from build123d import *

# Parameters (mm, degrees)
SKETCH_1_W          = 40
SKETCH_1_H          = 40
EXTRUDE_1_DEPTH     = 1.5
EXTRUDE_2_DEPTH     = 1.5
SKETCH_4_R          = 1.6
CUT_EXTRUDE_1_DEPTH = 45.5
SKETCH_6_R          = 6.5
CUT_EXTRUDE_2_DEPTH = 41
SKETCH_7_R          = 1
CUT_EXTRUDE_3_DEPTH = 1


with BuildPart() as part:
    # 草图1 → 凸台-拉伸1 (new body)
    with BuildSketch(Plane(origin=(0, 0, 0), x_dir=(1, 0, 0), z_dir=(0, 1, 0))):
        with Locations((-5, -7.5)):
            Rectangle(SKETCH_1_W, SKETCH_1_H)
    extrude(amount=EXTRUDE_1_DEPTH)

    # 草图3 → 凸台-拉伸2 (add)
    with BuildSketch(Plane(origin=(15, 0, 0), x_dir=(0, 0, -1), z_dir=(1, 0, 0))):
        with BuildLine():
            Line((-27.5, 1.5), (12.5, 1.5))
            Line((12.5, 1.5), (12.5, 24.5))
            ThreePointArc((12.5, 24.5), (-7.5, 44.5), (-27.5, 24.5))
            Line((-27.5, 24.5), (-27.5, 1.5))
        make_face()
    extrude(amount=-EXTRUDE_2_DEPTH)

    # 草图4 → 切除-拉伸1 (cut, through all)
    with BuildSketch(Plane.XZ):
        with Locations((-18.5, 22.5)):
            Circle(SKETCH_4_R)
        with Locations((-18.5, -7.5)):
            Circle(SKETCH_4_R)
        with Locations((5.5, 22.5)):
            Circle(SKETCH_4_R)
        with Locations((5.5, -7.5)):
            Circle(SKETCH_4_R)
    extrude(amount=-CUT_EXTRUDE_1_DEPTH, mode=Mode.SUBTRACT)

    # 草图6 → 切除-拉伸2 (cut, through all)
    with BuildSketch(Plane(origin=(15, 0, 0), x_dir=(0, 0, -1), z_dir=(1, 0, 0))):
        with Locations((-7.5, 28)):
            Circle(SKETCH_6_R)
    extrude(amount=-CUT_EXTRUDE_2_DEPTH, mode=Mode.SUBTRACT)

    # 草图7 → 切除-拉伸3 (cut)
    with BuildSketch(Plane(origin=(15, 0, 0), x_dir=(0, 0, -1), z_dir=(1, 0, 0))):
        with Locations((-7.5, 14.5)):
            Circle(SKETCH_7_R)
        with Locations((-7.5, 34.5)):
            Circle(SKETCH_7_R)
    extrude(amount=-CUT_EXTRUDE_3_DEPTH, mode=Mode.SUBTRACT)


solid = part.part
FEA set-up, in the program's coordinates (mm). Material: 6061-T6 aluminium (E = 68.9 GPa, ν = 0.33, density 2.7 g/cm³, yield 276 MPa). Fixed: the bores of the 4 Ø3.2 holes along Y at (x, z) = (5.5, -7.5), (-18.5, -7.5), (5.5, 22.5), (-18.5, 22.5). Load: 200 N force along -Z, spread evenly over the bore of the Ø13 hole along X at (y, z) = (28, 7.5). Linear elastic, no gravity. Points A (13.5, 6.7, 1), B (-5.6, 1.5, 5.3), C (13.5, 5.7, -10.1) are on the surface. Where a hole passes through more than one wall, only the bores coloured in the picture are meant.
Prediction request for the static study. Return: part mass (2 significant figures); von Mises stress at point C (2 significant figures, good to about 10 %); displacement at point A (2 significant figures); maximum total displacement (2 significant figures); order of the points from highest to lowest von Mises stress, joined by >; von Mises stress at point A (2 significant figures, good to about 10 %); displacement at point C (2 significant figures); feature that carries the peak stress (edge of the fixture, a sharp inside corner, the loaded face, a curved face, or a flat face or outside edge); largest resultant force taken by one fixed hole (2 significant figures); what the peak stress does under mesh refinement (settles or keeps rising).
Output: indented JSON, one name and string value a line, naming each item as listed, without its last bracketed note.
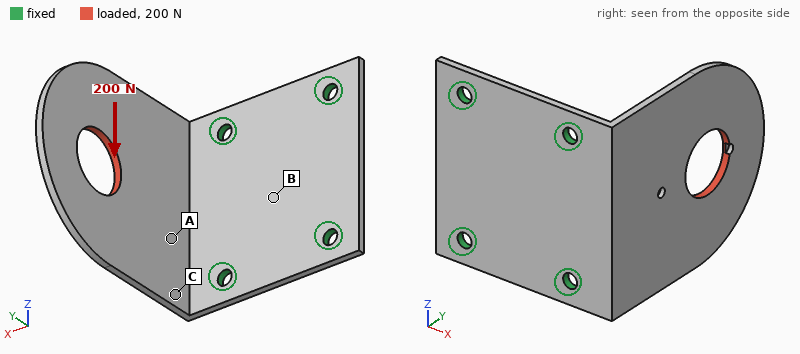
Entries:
{
  "part mass": "12 g",
  "von Mises stress at point C": "62 MPa",
  "displacement at point A": "0.051 mm",
  "maximum total displacement": "0.25 mm",
  "order of the points from highest to lowest von Mises stress, joined by >": "C > A > B",
  "von Mises stress at point A": "38 MPa",
  "displacement at point C": "0.10 mm",
  "feature that carries the peak stress": "edge of the fixture",
  "largest resultant force taken by one fixed hole": "210 N",
  "what the peak stress does under mesh refinement": "keeps rising"
}
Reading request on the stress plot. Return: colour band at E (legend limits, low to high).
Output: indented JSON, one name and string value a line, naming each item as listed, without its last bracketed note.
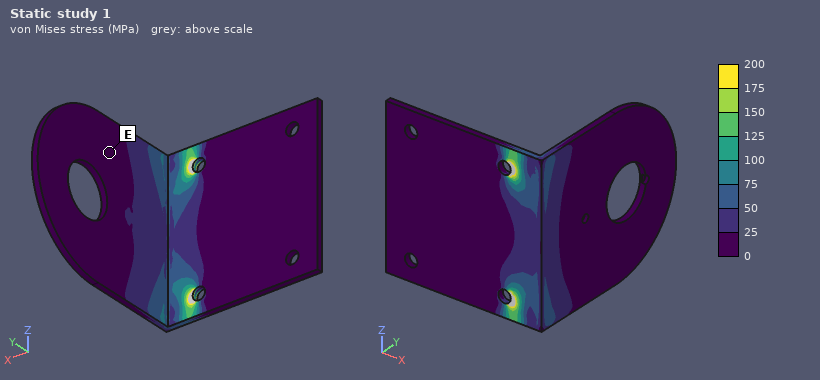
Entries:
{
  "colour band at E": "0 to 25 MPa"
}
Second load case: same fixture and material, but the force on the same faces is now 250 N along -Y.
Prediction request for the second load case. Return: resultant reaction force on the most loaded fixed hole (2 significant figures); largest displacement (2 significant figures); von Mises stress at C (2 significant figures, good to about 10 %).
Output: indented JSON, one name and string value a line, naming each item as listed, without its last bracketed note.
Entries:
{
  "resultant reaction force on the most loaded fixed hole": "130 N",
  "largest displacement": "0.51 mm",
  "von Mises stress at C": "16 MPa"
}
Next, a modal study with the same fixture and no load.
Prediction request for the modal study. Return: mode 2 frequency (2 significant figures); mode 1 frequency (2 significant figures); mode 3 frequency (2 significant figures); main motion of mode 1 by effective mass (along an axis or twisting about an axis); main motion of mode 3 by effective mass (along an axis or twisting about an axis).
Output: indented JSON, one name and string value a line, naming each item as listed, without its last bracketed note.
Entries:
{
  "mode 2 frequency": "1800 Hz",
  "mode 1 frequency": "610 Hz",
  "mode 3 frequency": "2900 Hz",
  "main motion of mode 1 by effective mass": "along X",
  "main motion of mode 3 by effective mass": "along Z"
}
